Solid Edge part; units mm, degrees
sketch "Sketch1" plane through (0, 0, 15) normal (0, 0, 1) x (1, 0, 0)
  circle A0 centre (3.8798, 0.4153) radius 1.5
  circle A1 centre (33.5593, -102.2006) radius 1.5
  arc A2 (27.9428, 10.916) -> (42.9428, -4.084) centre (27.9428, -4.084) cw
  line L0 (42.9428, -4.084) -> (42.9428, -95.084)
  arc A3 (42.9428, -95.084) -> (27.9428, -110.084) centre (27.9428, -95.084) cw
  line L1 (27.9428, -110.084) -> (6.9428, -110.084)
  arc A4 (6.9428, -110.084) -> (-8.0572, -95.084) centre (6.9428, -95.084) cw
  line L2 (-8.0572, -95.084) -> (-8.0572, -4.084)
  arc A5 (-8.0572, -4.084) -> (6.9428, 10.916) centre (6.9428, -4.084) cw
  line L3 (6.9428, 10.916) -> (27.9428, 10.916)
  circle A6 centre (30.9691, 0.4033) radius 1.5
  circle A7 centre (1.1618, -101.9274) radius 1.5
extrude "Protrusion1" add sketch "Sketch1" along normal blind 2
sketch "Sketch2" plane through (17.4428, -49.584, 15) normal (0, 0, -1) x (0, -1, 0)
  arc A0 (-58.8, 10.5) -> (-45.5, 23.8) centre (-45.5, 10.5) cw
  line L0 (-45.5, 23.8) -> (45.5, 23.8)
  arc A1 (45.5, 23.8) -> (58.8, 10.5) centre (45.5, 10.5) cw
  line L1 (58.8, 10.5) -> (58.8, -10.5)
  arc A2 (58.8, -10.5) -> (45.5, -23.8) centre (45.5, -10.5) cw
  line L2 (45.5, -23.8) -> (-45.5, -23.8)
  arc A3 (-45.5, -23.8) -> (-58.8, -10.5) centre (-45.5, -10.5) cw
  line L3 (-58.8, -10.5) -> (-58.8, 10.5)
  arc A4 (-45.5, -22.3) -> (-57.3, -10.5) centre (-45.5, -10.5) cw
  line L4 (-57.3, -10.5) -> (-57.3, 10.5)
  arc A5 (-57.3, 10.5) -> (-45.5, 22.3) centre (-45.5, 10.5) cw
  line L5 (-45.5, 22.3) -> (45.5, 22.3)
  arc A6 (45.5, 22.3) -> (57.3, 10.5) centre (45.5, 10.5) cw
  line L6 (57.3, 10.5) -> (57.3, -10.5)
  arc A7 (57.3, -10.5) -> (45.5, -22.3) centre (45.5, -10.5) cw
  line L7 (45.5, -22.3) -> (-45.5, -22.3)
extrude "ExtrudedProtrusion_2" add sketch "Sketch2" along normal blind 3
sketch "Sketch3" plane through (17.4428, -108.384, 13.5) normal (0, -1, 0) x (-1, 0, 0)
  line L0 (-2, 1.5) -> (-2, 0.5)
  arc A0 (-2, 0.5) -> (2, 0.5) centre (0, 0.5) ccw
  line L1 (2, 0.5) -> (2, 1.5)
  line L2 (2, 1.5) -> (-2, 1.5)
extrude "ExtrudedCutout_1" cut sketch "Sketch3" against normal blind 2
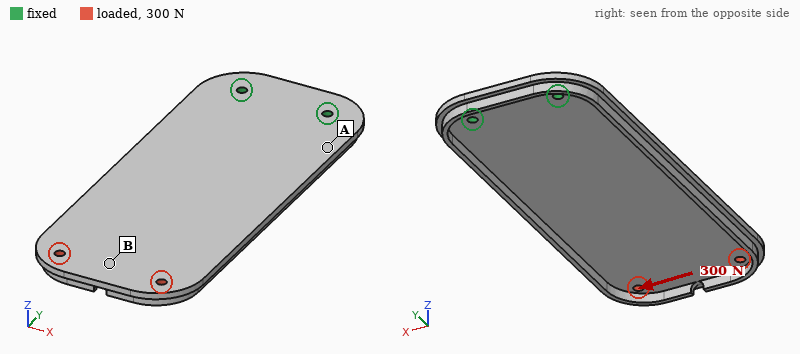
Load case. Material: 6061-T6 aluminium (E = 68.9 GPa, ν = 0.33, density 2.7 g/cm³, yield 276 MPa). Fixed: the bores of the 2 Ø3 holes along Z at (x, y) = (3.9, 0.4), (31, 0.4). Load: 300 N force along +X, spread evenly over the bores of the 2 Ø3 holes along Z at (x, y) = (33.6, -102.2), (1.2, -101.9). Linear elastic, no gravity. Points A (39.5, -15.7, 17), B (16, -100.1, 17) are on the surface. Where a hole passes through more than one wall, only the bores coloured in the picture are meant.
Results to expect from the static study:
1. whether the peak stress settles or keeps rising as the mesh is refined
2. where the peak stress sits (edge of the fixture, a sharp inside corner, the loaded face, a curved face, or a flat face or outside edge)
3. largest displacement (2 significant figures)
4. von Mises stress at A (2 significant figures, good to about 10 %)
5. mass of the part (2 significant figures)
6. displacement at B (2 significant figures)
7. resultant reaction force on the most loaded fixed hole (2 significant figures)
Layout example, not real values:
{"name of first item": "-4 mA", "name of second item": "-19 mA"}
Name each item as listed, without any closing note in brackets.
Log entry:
{"whether the peak stress settles or keeps rising as the mesh is refined": "keeps rising", "where the peak stress sits": "edge of the fixture", "largest displacement": "0.12 mm", "von Mises stress at A": "22 MPa", "mass of the part": "36 g", "displacement at B": "0.10 mm", "resultant reaction force on the most loaded fixed hole": "1.1 kN"}
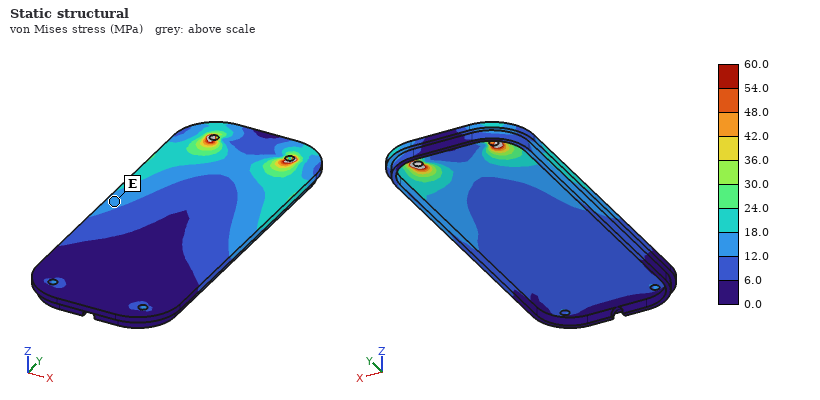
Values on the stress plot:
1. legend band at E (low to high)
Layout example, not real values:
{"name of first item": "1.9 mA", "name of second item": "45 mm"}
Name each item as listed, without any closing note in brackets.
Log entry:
{"legend band at E": "12.0 to 18.0 MPa"}
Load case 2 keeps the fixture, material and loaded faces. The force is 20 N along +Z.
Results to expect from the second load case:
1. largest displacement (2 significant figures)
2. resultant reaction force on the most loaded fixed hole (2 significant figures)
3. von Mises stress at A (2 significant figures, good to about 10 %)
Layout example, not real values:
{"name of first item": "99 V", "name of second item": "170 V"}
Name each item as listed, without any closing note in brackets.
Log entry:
{"largest displacement": "1.5 mm", "resultant reaction force on the most loaded fixed hole": "32 N", "von Mises stress at A": "24 MPa"}
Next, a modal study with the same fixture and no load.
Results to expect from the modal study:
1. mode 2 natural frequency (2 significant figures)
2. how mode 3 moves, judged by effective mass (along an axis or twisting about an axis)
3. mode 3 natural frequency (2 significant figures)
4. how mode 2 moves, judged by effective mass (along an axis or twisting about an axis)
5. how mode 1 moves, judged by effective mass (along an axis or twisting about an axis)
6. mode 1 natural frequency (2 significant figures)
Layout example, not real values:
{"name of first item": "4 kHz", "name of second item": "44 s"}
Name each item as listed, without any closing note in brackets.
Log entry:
{"mode 2 natural frequency": "650 Hz", "how mode 3 moves, judged by effective mass": "along Z", "mode 3 natural frequency": "1200 Hz", "how mode 2 moves, judged by effective mass": "twisting about Y", "how mode 1 moves, judged by effective mass": "along Z", "mode 1 natural frequency": "190 Hz"}
